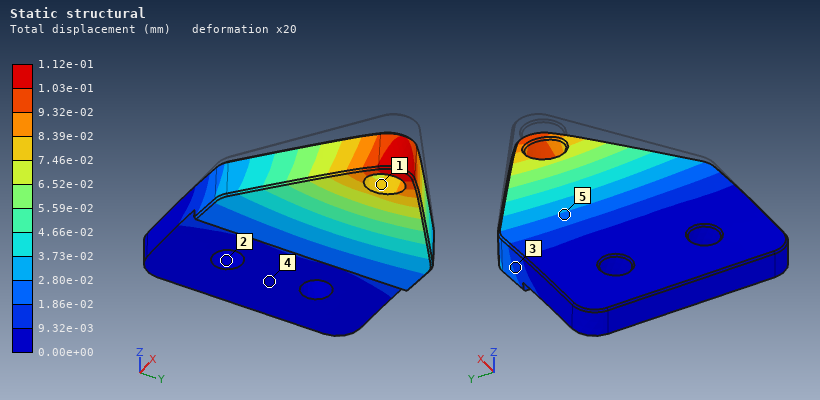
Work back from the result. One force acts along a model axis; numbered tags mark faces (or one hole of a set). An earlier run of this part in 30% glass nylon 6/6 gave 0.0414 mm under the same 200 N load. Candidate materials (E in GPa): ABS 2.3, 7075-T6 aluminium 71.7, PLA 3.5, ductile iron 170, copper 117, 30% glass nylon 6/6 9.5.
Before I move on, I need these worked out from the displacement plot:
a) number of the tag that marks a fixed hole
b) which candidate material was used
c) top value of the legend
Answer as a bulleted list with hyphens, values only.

- 2
- PLA
- 1.12e-01 mm
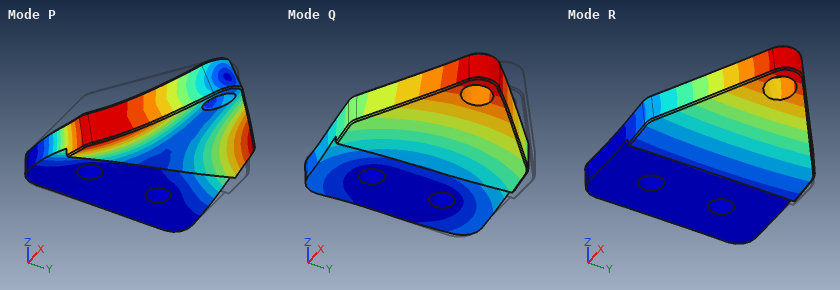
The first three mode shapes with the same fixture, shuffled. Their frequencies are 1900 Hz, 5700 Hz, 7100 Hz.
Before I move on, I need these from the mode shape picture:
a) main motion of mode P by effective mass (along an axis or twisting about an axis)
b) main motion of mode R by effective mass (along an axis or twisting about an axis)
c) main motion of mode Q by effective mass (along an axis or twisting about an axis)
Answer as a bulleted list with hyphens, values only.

- twisting about X
- along Z
- along Y
